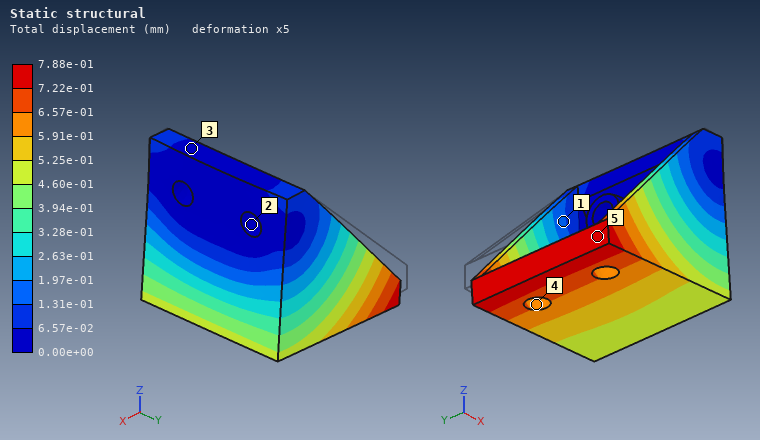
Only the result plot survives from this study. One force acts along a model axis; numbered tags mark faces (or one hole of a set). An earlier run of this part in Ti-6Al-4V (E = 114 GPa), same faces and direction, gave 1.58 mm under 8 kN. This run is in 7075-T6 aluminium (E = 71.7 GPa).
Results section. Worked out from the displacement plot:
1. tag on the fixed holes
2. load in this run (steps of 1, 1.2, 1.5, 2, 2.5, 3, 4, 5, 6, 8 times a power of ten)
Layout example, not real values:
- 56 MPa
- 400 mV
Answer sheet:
- 2
- 2.5 kN
